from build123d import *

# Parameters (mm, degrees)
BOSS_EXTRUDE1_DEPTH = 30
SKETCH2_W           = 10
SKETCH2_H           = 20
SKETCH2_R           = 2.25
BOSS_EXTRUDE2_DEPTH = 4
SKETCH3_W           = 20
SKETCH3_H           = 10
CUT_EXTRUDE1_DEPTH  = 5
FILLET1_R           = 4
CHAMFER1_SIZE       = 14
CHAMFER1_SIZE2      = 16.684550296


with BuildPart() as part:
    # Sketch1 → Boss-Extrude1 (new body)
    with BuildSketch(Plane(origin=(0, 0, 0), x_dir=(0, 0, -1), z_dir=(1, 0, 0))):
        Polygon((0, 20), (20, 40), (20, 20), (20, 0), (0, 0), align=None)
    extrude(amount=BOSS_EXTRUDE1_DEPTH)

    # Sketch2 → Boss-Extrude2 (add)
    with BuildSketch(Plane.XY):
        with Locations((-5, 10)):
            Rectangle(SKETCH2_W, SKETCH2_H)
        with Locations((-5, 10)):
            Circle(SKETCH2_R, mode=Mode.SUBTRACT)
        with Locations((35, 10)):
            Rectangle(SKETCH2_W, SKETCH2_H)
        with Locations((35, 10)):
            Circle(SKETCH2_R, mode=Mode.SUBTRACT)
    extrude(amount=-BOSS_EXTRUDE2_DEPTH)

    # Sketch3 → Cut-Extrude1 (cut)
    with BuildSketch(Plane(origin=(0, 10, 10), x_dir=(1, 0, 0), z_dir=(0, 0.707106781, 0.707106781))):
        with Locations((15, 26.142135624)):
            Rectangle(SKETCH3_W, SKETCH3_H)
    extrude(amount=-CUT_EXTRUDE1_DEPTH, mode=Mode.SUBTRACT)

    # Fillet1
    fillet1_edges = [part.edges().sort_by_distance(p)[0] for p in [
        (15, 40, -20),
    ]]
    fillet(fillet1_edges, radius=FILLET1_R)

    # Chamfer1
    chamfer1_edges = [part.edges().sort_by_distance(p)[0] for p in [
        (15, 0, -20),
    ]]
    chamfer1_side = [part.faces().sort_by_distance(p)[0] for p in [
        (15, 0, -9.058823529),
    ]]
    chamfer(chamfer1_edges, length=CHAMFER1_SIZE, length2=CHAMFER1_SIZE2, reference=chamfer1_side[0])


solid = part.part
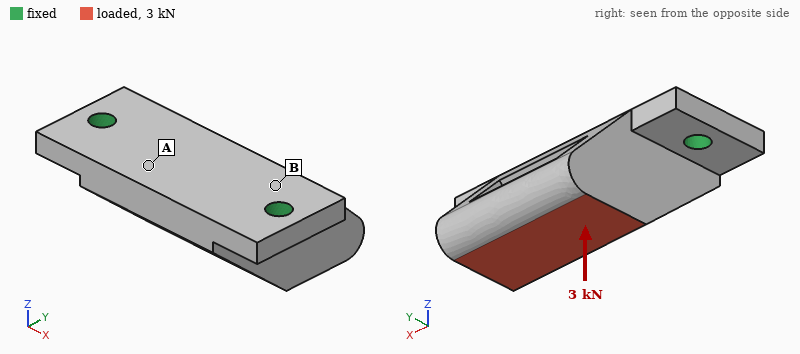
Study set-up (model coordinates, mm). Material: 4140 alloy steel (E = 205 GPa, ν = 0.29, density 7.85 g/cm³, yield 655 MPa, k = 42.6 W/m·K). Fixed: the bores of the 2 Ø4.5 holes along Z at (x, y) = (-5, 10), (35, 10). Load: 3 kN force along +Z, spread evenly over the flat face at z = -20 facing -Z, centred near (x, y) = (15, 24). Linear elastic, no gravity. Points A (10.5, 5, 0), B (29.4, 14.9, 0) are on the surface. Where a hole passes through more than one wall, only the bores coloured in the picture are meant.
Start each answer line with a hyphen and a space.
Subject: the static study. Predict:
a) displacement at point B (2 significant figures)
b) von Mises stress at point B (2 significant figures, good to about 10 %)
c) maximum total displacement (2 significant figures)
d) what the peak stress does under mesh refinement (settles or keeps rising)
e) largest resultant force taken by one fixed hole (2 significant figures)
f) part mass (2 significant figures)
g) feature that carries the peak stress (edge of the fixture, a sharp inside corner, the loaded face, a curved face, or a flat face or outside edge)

- 17 µm
- 130 MPa
- 97 µm
- keeps rising
- 1.7 kN
- 110 g
- edge of the fixture
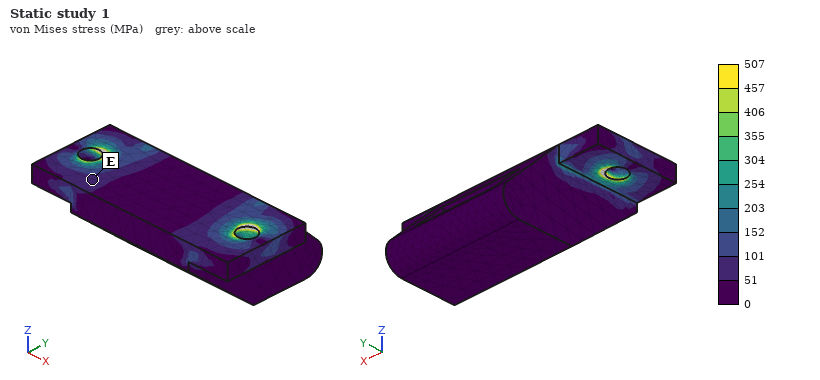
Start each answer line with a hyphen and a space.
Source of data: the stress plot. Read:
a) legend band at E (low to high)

- 51 to 101 MPa
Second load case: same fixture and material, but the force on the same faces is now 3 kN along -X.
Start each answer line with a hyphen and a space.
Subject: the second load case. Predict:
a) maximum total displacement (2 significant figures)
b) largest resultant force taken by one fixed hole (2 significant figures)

- 12 µm
- 2.4 kN
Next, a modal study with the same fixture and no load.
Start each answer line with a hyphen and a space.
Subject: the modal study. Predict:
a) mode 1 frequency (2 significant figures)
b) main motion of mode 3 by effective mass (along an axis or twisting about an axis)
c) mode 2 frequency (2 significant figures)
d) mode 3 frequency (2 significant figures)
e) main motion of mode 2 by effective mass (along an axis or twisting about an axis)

- 3900 Hz
- along X
- 13 kHz
- 14 kHz
- along Z
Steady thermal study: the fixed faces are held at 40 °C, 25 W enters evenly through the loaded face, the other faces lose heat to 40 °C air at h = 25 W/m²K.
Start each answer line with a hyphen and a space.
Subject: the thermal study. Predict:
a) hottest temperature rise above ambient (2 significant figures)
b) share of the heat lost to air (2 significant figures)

- 57 K
- 13 %
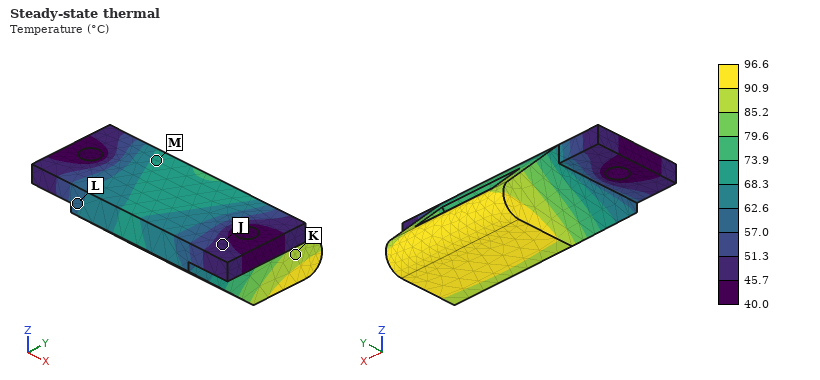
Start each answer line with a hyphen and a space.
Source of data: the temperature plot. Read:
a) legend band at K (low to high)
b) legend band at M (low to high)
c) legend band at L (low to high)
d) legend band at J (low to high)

- 85.2 to 90.9 °C
- 68.3 to 73.9 °C
- 57.0 to 62.6 °C
- 45.7 to 51.3 °C
